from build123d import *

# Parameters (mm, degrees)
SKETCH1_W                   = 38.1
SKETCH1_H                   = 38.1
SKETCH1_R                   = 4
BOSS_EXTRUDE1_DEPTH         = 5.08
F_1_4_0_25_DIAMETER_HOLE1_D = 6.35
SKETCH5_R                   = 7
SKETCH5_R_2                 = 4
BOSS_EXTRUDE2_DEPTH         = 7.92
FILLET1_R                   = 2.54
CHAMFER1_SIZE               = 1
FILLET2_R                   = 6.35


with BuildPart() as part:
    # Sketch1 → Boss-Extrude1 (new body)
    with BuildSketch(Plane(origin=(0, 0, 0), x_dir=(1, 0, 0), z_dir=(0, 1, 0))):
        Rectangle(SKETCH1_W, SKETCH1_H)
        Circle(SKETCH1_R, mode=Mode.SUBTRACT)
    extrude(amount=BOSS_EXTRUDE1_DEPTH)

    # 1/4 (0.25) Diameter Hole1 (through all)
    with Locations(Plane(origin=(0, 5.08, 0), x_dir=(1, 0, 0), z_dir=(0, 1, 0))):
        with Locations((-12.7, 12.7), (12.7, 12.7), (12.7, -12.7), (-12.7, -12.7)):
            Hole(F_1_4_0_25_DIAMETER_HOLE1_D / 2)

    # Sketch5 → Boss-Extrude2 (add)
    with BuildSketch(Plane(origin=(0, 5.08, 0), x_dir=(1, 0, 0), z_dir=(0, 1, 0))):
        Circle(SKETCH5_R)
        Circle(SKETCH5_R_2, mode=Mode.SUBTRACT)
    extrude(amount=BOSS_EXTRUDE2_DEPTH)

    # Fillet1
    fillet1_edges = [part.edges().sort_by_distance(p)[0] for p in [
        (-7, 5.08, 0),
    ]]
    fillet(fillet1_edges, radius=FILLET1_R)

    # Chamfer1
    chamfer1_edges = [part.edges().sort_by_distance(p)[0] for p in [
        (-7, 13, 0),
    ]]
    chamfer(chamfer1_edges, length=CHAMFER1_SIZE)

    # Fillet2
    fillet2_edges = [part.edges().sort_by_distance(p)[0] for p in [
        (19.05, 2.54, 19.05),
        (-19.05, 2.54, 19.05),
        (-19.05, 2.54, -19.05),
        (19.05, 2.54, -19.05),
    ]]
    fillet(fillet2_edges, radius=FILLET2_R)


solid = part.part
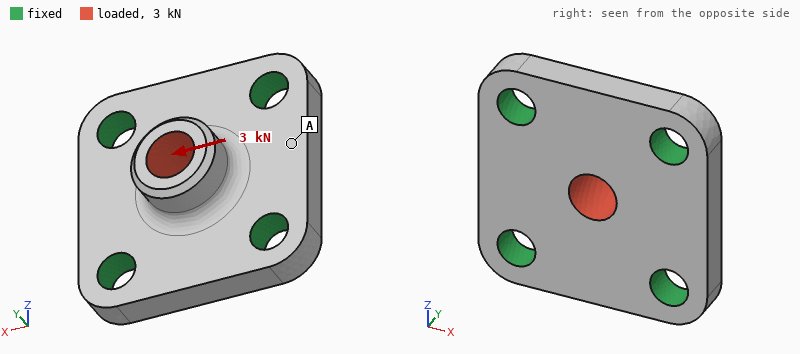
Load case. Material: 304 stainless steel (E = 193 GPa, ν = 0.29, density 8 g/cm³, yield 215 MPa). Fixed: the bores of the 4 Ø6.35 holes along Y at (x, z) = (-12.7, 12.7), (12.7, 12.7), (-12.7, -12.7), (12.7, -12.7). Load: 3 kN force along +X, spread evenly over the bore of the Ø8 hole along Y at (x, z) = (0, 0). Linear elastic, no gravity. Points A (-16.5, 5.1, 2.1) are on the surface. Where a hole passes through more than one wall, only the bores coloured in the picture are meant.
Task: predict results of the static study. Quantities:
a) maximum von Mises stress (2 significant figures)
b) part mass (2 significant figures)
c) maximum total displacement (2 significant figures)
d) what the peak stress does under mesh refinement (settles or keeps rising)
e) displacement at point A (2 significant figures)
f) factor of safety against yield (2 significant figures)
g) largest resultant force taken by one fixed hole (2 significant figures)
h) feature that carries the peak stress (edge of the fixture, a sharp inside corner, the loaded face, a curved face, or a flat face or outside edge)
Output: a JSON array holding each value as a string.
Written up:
["59 MPa", "57 g", "4.6 µm", "settles", "0.82 µm", "3.7", "870 N", "a curved face"]
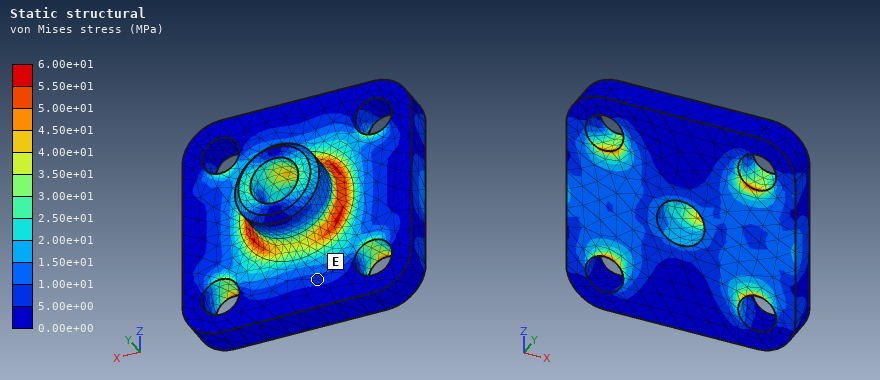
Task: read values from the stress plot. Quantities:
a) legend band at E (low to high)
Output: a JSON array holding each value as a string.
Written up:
["5.00e+00 to 1.00e+01 MPa"]
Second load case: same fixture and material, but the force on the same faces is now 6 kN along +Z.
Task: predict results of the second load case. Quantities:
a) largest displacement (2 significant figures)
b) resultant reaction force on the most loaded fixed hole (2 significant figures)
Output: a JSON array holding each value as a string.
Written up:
["9.2 µm", "1.7 kN"]
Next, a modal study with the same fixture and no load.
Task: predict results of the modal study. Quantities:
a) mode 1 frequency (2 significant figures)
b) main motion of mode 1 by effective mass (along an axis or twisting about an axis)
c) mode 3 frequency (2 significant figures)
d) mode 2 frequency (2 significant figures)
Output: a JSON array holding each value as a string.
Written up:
["30 kHz", "along Y", "38 kHz", "38 kHz"]
